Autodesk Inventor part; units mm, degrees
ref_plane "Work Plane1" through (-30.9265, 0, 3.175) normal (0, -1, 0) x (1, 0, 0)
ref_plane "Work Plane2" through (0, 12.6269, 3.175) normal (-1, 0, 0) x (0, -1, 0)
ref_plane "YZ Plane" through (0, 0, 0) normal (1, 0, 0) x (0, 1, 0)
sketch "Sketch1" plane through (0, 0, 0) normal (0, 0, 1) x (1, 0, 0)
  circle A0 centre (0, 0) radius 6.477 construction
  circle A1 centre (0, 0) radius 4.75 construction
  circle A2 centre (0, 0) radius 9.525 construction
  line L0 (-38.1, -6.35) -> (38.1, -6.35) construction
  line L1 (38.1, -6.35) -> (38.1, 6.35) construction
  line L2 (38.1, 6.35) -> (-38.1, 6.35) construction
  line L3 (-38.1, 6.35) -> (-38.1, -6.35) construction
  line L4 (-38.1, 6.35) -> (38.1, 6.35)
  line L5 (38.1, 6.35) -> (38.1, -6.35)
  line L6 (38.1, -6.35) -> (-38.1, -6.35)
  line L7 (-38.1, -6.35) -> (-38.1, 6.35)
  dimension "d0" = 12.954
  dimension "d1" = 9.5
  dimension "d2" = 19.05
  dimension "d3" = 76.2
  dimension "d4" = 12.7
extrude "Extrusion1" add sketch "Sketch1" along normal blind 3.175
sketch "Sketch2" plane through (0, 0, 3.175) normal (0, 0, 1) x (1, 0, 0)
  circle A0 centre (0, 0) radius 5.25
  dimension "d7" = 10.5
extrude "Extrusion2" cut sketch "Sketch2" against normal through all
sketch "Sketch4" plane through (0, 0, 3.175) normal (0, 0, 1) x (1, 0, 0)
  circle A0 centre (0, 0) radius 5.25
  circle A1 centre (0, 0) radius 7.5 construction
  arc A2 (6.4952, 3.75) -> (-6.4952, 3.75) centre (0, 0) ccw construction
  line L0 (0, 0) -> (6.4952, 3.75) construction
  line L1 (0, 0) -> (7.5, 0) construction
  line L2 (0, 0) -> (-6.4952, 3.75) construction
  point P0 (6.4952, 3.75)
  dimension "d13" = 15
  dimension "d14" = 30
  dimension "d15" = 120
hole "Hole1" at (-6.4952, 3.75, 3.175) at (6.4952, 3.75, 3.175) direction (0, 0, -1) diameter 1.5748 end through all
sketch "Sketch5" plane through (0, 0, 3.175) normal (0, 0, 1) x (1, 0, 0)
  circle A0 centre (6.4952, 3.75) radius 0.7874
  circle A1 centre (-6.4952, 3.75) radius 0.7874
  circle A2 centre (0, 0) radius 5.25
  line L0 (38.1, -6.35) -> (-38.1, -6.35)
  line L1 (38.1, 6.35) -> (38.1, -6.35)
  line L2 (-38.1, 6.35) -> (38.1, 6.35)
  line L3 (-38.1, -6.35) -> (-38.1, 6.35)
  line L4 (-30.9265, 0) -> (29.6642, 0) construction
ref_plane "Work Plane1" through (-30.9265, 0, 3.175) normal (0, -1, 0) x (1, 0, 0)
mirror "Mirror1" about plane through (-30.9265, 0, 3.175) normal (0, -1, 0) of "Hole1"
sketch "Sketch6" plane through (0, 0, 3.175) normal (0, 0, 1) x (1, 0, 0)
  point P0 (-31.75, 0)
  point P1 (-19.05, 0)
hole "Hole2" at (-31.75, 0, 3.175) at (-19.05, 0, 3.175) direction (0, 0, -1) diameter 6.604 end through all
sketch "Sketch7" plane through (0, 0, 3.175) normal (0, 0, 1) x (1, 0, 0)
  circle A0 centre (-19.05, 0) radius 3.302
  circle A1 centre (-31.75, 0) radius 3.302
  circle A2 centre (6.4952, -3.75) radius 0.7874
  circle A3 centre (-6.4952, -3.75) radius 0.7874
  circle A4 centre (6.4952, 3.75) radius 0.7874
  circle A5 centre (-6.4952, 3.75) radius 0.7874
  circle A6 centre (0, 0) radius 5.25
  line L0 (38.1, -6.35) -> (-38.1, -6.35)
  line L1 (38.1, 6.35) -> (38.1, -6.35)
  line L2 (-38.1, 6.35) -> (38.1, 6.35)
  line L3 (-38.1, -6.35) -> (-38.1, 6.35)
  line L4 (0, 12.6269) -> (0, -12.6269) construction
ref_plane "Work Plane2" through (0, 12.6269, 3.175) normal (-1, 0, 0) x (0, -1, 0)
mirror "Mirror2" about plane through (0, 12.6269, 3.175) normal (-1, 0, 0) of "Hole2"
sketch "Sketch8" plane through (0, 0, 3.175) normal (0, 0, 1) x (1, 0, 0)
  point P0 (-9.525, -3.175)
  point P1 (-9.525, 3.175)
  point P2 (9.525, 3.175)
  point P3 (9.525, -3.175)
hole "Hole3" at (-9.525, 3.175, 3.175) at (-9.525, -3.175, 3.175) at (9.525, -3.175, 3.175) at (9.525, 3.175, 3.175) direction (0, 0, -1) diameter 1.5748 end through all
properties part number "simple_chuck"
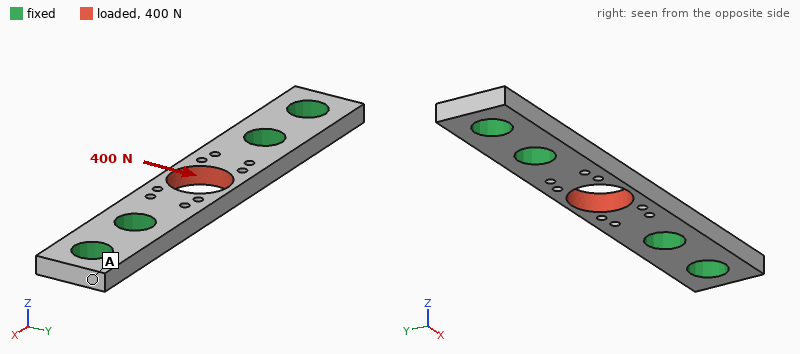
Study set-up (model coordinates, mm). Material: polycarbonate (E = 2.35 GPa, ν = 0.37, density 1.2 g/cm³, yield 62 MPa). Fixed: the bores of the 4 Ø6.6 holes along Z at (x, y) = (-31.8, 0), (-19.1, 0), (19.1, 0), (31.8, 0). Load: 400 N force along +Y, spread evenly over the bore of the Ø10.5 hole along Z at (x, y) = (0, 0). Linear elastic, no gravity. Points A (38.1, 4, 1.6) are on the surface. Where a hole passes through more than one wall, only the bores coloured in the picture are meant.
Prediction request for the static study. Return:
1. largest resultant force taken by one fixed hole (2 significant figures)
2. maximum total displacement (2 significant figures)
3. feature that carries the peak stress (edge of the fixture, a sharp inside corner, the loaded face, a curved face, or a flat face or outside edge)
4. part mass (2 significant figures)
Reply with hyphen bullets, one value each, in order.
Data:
- 220 N
- 0.26 mm
- a flat face or outside edge
- 2.8 g
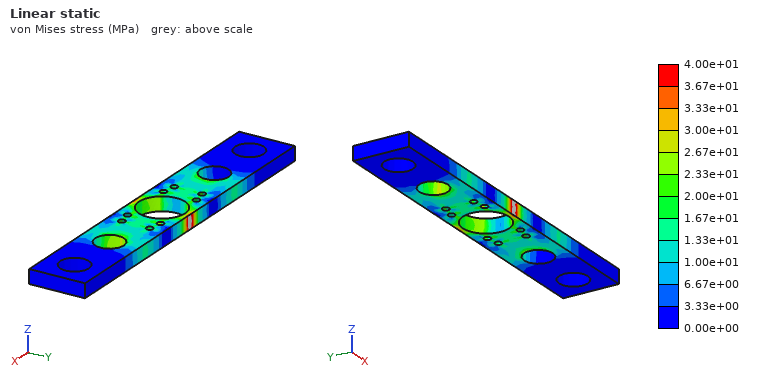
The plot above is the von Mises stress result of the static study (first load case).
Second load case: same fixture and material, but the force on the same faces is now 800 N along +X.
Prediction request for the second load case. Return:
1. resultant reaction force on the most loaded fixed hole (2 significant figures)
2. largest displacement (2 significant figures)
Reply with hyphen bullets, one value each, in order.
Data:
- 380 N
- 94 µm
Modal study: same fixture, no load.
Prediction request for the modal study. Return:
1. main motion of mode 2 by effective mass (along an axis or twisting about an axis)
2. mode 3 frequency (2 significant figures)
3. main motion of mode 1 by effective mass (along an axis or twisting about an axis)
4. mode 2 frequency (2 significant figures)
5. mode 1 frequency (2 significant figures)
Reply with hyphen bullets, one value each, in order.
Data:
- twisting about X
- 8800 Hz
- along Z
- 6600 Hz
- 4600 Hz
